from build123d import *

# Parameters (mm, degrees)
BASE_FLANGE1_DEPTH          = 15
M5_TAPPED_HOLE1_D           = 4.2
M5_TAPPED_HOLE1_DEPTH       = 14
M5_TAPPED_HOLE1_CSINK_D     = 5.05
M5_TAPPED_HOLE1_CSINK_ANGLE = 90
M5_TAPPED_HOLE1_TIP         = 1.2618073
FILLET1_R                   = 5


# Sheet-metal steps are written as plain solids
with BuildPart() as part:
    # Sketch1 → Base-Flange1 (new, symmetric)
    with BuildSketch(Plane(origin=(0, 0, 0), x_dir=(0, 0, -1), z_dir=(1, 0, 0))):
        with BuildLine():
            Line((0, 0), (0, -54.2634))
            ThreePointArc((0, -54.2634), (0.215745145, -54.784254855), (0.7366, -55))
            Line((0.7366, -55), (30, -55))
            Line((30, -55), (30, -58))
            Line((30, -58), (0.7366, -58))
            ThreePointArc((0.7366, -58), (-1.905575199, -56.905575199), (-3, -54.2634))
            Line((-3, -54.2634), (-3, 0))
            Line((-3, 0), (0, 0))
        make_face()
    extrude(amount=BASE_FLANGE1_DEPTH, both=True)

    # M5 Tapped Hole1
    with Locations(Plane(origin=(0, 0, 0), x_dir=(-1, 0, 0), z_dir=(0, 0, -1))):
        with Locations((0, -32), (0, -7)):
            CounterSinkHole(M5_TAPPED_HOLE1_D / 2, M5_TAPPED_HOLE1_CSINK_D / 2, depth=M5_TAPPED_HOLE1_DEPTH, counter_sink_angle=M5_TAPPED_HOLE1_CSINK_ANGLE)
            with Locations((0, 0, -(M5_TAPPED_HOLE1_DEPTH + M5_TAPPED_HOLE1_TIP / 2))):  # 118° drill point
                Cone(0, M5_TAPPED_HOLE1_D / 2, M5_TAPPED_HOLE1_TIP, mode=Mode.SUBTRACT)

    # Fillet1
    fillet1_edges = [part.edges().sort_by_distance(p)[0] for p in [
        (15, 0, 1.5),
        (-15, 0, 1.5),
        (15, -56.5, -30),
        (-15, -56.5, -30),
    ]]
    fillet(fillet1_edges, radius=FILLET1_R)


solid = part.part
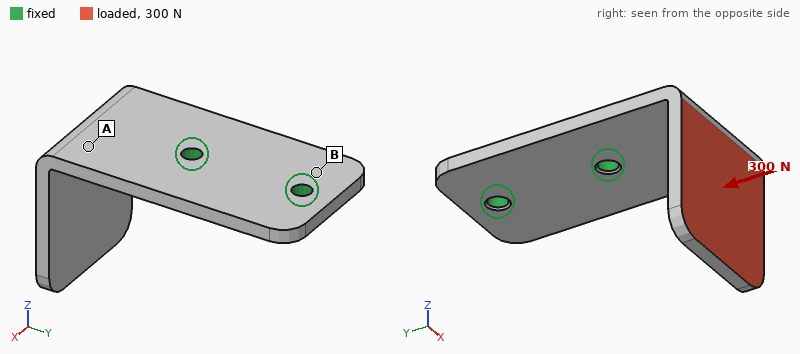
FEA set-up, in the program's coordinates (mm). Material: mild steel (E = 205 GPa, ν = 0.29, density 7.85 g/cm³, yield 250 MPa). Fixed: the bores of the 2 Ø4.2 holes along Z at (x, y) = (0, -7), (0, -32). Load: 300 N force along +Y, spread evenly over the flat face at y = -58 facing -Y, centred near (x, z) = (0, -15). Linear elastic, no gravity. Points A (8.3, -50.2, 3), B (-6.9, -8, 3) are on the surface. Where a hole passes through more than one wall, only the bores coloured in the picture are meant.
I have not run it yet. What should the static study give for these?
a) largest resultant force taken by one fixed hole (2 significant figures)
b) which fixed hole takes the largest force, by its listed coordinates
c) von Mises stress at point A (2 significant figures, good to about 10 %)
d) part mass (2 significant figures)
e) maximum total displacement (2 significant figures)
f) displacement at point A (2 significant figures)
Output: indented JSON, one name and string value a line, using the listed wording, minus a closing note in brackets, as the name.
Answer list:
{
  "largest resultant force taken by one fixed hole": "220 N",
  "which fixed hole takes the largest force, by its listed coordinates": "(0, -32)",
  "von Mises stress at point A": "98 MPa",
  "part mass": "60 g",
  "maximum total displacement": "0.38 mm",
  "displacement at point A": "0.064 mm"
}
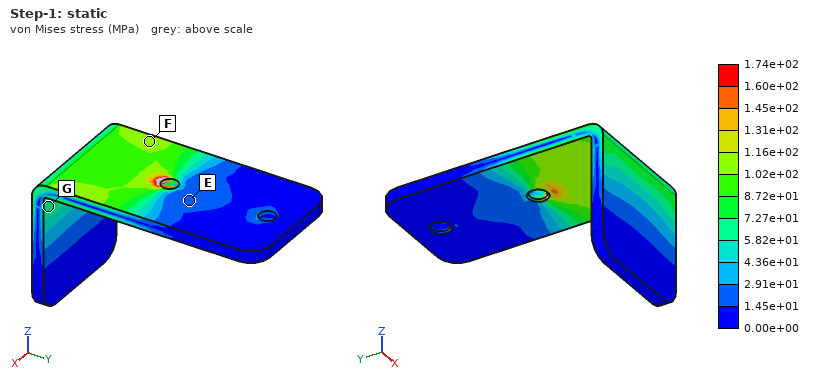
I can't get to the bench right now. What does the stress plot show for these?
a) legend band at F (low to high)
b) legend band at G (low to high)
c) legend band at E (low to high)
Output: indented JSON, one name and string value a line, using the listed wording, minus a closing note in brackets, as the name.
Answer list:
{
  "legend band at F": "1.02e+02 to 1.16e+02 MPa",
  "legend band at G": "5.82e+01 to 7.27e+01 MPa",
  "legend band at E": "1.45e+01 to 2.91e+01 MPa"
}
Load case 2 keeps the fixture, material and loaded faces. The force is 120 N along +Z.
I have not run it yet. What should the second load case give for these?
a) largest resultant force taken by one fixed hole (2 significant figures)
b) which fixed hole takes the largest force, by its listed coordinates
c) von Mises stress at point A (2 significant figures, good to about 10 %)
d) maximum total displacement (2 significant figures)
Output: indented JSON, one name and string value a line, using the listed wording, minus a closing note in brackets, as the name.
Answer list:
{
  "largest resultant force taken by one fixed hole": "160 N",
  "which fixed hole takes the largest force, by its listed coordinates": "(0, -32)",
  "von Mises stress at point A": "19 MPa",
  "maximum total displacement": "0.11 mm"
}
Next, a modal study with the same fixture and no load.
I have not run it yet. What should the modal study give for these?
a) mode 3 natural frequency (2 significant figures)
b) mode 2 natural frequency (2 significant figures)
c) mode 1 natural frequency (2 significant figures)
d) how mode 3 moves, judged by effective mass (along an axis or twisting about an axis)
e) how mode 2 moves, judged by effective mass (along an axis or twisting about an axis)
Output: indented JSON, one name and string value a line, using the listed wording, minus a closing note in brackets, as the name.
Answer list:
{
  "mode 3 natural frequency": "2900 Hz",
  "mode 2 natural frequency": "1600 Hz",
  "mode 1 natural frequency": "1100 Hz",
  "how mode 3 moves, judged by effective mass": "along Z",
  "how mode 2 moves, judged by effective mass": "along X"
}
